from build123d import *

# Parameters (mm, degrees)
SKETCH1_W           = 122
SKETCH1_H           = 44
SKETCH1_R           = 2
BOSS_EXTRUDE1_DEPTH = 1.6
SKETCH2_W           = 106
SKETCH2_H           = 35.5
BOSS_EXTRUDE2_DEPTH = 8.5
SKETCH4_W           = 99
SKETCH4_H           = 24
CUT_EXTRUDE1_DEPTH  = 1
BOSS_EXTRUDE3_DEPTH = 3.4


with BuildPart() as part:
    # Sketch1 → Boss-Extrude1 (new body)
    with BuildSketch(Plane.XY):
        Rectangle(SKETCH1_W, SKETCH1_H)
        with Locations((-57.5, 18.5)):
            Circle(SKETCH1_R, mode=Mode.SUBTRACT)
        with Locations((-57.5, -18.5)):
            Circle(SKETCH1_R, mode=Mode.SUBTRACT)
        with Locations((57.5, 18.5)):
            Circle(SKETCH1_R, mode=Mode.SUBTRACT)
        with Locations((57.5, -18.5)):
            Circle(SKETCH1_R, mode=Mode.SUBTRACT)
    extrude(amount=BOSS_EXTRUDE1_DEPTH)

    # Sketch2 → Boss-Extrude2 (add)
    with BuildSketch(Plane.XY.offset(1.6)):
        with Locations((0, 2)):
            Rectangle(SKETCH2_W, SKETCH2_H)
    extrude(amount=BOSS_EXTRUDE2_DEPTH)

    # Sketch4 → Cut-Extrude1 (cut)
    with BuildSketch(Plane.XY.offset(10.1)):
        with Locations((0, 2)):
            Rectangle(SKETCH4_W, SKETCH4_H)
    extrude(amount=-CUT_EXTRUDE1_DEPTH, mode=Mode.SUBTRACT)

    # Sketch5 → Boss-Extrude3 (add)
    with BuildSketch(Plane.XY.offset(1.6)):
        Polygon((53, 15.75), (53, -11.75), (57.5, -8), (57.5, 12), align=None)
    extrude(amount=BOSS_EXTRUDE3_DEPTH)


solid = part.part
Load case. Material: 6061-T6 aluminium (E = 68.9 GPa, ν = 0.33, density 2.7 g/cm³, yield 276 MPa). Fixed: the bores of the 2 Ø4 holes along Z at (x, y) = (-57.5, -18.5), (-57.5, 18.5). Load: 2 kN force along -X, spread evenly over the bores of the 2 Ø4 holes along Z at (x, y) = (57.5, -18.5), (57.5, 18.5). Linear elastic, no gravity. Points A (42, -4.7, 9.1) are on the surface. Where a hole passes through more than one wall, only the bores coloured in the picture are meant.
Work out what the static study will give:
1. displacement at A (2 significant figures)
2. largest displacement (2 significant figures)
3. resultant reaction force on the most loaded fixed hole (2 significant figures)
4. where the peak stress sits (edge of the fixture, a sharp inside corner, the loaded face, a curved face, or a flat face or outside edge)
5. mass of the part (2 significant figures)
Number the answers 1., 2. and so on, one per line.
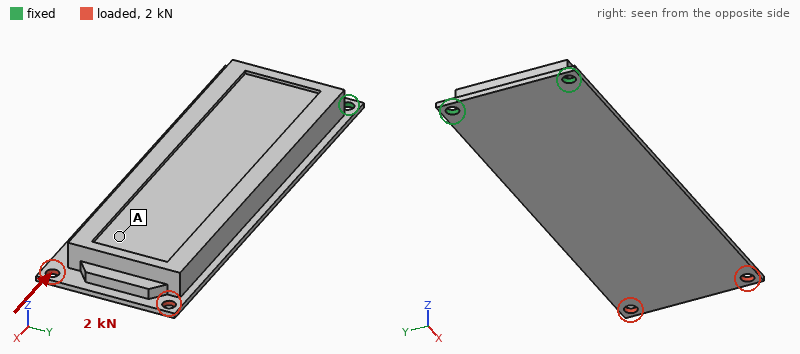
1. 0.21 mm
2. 0.30 mm
3. 1.0 kN
4. the loaded face
5. 100 g
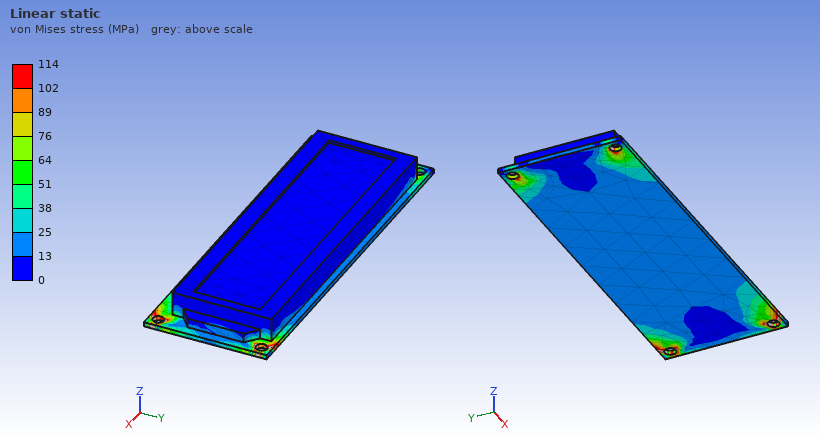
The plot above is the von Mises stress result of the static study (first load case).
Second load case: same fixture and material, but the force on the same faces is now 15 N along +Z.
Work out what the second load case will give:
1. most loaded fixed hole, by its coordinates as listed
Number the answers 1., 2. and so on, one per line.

1. (-57.5, -18.5)
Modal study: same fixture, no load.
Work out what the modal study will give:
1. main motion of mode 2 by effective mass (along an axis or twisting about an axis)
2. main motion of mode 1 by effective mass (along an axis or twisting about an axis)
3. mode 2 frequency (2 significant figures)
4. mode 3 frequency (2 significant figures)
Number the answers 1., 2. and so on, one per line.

1. along Y
2. along Z
3. 1600 Hz
4. 2400 Hz
